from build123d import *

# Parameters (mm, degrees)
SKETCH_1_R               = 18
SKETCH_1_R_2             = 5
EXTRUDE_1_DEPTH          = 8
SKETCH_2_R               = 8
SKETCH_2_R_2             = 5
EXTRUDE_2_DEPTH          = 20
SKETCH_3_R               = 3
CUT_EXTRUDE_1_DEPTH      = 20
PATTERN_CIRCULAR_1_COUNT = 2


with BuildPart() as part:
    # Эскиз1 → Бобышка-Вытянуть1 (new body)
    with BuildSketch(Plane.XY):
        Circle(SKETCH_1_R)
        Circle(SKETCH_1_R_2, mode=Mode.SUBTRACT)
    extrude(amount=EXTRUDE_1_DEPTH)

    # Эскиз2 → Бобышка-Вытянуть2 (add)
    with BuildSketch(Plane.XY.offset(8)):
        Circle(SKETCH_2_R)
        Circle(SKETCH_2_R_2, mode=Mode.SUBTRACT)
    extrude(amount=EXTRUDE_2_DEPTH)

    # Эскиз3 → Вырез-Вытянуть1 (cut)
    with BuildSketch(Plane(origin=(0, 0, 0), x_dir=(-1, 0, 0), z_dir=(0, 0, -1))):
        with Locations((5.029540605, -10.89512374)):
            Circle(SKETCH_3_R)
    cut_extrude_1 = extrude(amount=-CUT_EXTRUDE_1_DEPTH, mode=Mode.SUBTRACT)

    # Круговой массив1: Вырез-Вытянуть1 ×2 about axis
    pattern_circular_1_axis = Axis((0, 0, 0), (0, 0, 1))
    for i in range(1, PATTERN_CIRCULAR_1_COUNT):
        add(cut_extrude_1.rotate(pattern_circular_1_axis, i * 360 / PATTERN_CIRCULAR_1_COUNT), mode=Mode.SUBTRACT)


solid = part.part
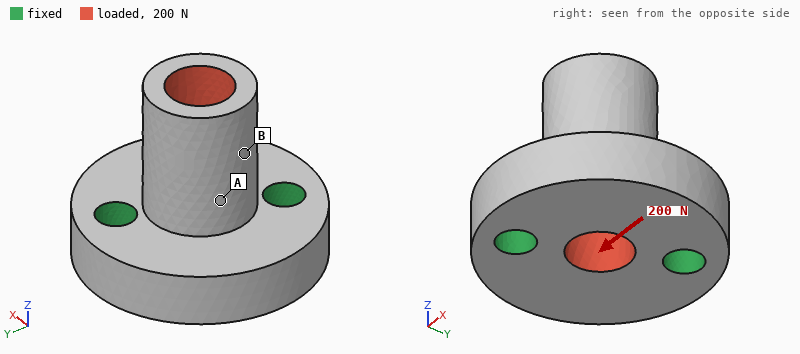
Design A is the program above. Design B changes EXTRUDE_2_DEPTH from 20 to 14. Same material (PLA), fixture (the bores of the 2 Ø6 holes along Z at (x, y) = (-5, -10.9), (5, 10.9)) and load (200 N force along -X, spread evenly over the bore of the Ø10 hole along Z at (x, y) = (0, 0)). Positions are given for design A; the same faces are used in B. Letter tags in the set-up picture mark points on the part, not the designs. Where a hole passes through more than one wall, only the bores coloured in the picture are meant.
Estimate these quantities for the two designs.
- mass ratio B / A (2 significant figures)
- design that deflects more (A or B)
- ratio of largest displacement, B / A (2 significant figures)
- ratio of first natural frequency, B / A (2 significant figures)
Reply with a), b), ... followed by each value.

a) 0.92
b) A
c) 0.52
d) 1.3
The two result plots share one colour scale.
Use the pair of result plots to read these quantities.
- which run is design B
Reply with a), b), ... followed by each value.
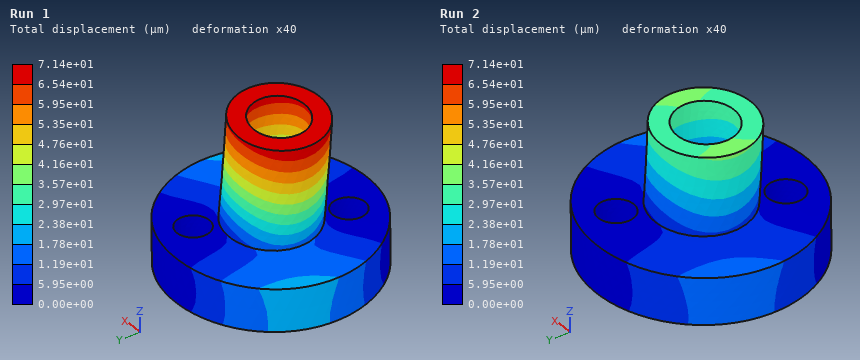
a) Run 2
